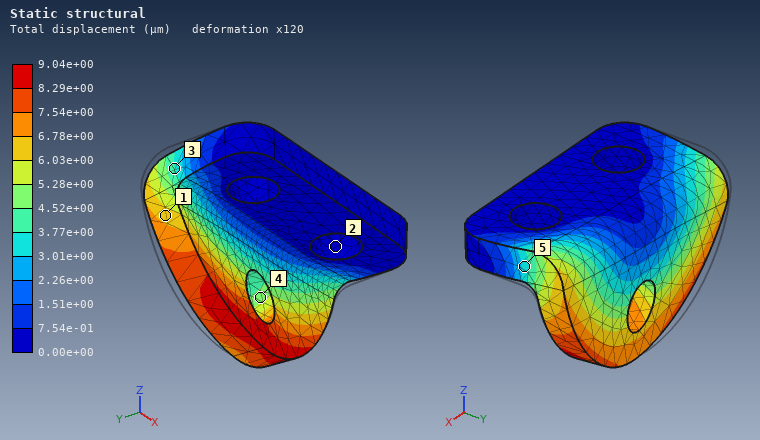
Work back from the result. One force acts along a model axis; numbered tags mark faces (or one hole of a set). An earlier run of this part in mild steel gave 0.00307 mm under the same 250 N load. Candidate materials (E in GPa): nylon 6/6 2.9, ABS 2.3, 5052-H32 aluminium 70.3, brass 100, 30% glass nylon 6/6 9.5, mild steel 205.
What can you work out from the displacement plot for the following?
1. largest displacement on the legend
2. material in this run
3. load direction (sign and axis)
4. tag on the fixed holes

9.04e+00 µm
5052-H32 aluminium
+X
2
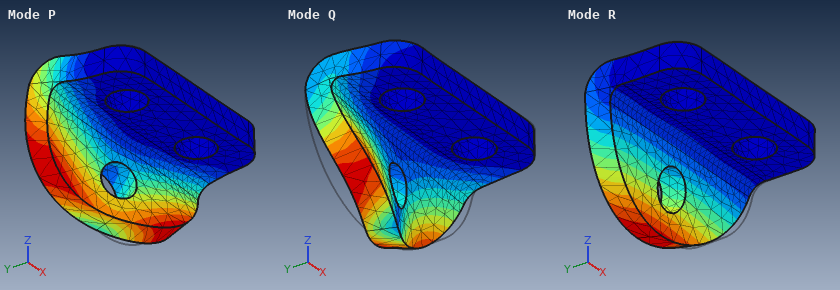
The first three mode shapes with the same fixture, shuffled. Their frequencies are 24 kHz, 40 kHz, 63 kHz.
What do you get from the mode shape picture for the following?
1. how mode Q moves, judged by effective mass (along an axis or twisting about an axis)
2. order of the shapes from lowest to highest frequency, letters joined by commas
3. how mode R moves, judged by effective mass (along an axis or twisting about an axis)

along X
R, P, Q
along Y
